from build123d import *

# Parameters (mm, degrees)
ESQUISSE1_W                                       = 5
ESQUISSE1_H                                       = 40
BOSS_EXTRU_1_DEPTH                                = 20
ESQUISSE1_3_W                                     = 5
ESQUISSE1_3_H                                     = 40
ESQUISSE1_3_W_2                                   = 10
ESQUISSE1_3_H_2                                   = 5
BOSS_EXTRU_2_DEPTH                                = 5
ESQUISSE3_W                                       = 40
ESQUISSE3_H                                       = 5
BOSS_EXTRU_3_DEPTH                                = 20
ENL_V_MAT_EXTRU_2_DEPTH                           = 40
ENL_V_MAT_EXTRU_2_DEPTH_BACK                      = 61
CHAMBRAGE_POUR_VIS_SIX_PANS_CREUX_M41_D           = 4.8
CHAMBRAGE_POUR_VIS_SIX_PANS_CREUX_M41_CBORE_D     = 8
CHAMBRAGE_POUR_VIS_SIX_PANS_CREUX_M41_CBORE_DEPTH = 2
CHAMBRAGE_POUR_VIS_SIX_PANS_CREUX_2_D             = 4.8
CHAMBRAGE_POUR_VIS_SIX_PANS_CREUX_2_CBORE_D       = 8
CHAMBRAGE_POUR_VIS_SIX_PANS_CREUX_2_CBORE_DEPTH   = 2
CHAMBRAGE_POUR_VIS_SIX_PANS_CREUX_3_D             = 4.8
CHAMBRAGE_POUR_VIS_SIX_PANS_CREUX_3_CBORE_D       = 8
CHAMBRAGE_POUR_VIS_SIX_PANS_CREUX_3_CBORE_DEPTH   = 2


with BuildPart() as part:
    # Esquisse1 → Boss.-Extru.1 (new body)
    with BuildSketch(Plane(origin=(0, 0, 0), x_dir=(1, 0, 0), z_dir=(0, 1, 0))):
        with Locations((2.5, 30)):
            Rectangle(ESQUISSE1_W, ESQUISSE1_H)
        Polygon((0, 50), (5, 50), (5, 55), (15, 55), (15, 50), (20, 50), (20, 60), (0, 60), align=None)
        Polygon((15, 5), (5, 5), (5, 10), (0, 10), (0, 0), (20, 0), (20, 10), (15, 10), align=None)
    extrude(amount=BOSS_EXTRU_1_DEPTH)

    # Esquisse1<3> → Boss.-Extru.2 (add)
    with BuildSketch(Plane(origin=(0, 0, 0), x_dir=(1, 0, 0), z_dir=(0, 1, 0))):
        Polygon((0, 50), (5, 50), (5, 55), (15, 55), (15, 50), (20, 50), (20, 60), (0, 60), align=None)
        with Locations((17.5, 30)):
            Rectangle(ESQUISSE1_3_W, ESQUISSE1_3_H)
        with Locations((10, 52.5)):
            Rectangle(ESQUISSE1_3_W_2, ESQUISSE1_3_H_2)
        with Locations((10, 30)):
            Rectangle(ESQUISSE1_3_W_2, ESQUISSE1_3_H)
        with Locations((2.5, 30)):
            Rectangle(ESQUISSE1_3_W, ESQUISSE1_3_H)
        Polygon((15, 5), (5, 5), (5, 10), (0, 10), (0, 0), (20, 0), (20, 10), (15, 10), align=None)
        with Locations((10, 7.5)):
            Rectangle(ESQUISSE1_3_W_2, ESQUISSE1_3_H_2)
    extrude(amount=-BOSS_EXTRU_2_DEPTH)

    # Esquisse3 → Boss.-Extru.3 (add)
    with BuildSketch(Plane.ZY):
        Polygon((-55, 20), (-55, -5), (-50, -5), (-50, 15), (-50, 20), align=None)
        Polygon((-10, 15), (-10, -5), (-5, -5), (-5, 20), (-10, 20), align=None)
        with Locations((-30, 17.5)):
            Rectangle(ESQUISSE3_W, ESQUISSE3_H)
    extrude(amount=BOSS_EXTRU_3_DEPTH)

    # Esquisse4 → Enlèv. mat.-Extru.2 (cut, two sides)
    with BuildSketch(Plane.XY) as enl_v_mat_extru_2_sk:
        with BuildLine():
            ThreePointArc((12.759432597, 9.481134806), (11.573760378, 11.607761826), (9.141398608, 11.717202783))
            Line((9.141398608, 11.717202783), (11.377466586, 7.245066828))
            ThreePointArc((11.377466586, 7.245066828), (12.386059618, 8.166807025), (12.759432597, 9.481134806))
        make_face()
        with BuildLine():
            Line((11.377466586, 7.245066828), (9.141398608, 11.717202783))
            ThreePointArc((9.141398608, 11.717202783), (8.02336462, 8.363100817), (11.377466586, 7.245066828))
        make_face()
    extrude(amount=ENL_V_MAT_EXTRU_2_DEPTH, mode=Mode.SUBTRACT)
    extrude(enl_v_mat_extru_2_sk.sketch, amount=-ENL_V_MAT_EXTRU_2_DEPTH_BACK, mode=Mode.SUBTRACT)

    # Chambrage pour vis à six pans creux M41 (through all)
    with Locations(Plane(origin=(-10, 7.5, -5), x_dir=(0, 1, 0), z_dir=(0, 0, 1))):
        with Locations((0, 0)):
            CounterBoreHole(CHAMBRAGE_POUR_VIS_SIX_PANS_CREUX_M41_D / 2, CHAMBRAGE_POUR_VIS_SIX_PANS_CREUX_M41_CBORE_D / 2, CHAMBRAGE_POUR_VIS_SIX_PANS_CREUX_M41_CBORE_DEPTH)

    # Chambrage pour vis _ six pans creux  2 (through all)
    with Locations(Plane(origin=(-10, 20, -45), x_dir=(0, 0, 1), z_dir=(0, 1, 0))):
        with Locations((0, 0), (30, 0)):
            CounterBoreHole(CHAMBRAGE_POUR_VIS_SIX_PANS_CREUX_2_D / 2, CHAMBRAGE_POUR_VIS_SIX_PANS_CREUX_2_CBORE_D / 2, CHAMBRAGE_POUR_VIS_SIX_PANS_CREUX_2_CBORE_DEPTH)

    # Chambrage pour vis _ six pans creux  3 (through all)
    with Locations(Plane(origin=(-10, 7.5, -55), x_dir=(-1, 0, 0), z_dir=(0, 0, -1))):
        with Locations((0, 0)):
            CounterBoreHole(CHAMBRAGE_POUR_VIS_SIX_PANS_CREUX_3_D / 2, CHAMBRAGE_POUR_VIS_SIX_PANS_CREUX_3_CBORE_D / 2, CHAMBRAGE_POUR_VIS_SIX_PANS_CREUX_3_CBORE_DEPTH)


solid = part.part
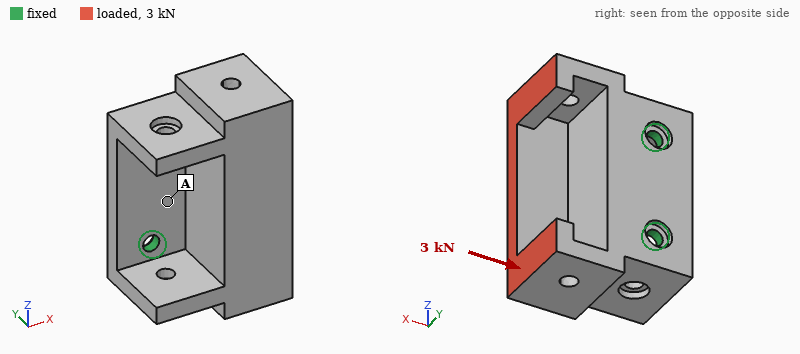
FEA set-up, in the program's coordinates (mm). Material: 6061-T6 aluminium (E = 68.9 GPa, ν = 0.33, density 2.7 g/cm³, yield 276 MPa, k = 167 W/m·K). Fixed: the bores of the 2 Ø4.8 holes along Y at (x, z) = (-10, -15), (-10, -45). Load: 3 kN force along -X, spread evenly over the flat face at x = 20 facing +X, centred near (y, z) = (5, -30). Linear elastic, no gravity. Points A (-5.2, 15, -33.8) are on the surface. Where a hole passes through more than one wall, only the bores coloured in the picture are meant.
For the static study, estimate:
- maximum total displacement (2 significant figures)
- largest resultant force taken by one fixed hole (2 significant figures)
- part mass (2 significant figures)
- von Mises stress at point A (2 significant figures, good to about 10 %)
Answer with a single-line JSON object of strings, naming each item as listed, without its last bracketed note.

{"maximum total displacement": "0.29 mm", "largest resultant force taken by one fixed hole": "1.5 kN", "part mass": "65 g", "von Mises stress at point A": "51 MPa"}
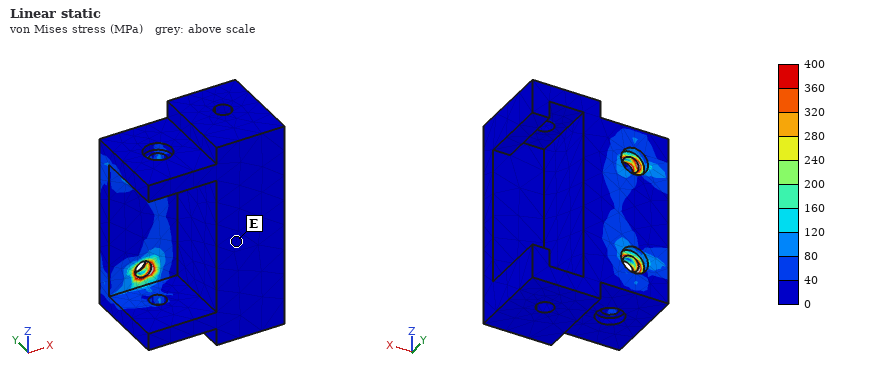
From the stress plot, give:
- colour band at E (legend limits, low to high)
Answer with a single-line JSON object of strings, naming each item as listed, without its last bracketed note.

{"colour band at E": "0 to 40 MPa"}
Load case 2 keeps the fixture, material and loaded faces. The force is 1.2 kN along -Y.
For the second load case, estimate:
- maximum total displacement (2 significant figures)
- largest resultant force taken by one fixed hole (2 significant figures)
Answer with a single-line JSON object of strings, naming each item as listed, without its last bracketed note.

{"maximum total displacement": "0.30 mm", "largest resultant force taken by one fixed hole": "700 N"}
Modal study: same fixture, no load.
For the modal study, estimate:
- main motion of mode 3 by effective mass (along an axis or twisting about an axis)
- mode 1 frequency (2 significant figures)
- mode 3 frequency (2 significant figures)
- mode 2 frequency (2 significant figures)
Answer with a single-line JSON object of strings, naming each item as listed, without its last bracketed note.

{"main motion of mode 3 by effective mass": "along Z", "mode 1 frequency": "2100 Hz", "mode 3 frequency": "6900 Hz", "mode 2 frequency": "3500 Hz"}
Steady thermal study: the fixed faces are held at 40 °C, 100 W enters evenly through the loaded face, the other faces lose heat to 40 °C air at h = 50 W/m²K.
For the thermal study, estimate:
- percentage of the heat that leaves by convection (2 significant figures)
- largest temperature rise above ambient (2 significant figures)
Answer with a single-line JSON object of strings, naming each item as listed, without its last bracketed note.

{"percentage of the heat that leaves by convection": "17 %", "largest temperature rise above ambient": "62 K"}
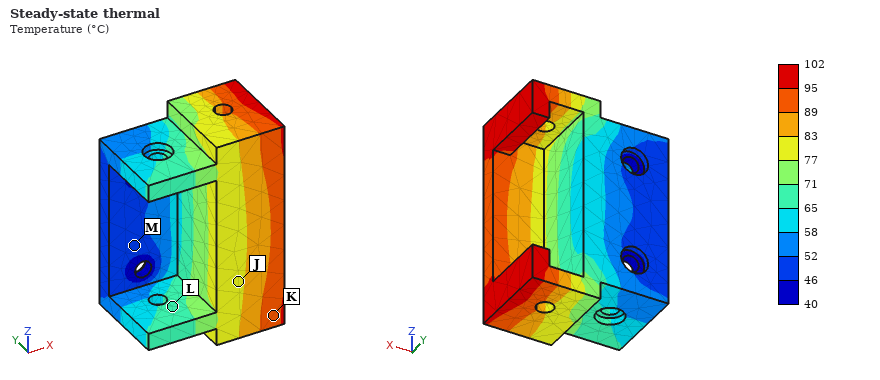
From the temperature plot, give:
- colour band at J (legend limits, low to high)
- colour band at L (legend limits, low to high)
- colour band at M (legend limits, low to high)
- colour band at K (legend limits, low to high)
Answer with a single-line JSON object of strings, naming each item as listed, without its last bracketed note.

{"colour band at J": "77 to 83 °C", "colour band at L": "65 to 71 °C", "colour band at M": "46 to 52 °C", "colour band at K": "89 to 95 °C"}
